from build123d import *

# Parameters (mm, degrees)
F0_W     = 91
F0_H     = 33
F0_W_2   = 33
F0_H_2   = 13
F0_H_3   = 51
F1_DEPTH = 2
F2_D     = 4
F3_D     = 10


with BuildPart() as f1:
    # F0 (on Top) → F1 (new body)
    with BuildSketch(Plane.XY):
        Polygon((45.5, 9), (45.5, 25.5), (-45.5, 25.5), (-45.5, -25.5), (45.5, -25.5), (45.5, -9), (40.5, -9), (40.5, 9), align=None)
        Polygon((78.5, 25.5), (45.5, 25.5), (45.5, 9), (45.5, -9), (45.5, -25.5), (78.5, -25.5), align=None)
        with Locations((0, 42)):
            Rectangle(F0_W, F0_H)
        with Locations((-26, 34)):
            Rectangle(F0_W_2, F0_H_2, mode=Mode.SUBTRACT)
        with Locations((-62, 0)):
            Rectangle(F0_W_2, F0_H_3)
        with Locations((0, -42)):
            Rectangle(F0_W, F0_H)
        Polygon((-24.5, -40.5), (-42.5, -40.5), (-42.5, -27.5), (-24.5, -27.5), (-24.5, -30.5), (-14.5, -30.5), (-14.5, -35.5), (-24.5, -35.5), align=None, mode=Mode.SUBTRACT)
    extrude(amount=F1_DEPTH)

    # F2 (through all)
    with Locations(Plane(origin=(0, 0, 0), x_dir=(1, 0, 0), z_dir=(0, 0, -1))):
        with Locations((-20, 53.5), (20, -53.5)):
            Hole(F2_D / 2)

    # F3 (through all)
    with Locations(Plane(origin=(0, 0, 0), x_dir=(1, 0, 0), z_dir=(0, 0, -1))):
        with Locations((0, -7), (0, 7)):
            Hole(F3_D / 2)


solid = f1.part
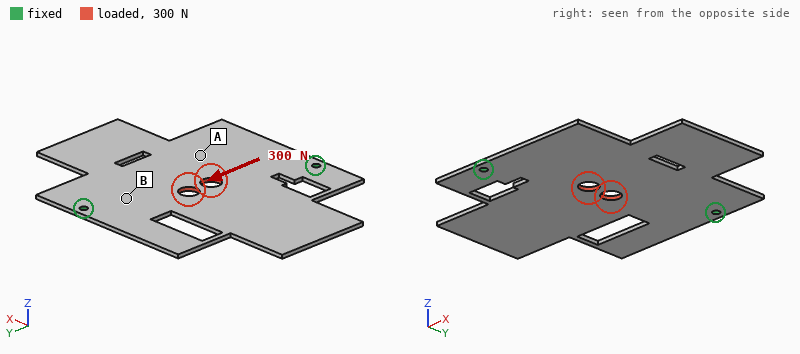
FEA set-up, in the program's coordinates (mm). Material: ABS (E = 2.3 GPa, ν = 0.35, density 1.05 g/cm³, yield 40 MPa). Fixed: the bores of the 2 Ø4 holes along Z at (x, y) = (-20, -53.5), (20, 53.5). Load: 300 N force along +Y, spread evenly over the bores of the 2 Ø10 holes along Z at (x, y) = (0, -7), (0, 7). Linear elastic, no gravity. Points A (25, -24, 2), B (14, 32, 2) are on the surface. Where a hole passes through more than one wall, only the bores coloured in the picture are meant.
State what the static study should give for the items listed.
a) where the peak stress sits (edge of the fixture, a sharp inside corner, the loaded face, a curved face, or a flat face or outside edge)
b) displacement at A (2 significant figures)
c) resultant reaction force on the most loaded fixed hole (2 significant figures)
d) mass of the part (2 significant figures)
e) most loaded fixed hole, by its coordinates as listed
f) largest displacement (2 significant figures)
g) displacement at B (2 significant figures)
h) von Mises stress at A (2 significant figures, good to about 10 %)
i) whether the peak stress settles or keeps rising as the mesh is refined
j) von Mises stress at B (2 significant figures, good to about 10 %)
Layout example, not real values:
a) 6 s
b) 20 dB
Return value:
a) edge of the fixture
b) 0.076 mm
c) 190 N
d) 27 g
e) (20, 53.5)
f) 0.13 mm
g) 0.050 mm
h) 0.82 MPa
i) keeps rising
j) 3.0 MPa
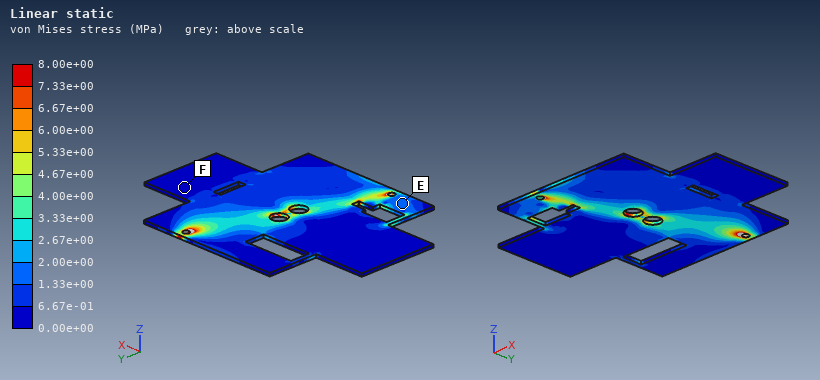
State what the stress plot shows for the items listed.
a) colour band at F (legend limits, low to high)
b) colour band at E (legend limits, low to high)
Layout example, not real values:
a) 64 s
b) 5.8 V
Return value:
a) 0.00e+00 to 6.67e-01 MPa
b) 1.33e+00 to 2.00e+00 MPa
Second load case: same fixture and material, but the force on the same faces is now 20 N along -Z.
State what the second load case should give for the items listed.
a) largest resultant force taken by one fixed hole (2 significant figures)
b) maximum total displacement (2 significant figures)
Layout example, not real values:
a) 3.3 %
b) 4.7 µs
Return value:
a) 10 N
b) 2.2 mm
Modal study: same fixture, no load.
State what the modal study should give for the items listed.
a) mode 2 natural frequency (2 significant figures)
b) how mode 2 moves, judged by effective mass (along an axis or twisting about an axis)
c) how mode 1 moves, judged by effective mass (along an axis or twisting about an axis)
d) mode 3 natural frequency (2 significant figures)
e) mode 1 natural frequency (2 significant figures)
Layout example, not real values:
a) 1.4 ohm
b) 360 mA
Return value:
a) 90 Hz
b) along Z
c) twisting about Y
d) 190 Hz
e) 61 Hz
